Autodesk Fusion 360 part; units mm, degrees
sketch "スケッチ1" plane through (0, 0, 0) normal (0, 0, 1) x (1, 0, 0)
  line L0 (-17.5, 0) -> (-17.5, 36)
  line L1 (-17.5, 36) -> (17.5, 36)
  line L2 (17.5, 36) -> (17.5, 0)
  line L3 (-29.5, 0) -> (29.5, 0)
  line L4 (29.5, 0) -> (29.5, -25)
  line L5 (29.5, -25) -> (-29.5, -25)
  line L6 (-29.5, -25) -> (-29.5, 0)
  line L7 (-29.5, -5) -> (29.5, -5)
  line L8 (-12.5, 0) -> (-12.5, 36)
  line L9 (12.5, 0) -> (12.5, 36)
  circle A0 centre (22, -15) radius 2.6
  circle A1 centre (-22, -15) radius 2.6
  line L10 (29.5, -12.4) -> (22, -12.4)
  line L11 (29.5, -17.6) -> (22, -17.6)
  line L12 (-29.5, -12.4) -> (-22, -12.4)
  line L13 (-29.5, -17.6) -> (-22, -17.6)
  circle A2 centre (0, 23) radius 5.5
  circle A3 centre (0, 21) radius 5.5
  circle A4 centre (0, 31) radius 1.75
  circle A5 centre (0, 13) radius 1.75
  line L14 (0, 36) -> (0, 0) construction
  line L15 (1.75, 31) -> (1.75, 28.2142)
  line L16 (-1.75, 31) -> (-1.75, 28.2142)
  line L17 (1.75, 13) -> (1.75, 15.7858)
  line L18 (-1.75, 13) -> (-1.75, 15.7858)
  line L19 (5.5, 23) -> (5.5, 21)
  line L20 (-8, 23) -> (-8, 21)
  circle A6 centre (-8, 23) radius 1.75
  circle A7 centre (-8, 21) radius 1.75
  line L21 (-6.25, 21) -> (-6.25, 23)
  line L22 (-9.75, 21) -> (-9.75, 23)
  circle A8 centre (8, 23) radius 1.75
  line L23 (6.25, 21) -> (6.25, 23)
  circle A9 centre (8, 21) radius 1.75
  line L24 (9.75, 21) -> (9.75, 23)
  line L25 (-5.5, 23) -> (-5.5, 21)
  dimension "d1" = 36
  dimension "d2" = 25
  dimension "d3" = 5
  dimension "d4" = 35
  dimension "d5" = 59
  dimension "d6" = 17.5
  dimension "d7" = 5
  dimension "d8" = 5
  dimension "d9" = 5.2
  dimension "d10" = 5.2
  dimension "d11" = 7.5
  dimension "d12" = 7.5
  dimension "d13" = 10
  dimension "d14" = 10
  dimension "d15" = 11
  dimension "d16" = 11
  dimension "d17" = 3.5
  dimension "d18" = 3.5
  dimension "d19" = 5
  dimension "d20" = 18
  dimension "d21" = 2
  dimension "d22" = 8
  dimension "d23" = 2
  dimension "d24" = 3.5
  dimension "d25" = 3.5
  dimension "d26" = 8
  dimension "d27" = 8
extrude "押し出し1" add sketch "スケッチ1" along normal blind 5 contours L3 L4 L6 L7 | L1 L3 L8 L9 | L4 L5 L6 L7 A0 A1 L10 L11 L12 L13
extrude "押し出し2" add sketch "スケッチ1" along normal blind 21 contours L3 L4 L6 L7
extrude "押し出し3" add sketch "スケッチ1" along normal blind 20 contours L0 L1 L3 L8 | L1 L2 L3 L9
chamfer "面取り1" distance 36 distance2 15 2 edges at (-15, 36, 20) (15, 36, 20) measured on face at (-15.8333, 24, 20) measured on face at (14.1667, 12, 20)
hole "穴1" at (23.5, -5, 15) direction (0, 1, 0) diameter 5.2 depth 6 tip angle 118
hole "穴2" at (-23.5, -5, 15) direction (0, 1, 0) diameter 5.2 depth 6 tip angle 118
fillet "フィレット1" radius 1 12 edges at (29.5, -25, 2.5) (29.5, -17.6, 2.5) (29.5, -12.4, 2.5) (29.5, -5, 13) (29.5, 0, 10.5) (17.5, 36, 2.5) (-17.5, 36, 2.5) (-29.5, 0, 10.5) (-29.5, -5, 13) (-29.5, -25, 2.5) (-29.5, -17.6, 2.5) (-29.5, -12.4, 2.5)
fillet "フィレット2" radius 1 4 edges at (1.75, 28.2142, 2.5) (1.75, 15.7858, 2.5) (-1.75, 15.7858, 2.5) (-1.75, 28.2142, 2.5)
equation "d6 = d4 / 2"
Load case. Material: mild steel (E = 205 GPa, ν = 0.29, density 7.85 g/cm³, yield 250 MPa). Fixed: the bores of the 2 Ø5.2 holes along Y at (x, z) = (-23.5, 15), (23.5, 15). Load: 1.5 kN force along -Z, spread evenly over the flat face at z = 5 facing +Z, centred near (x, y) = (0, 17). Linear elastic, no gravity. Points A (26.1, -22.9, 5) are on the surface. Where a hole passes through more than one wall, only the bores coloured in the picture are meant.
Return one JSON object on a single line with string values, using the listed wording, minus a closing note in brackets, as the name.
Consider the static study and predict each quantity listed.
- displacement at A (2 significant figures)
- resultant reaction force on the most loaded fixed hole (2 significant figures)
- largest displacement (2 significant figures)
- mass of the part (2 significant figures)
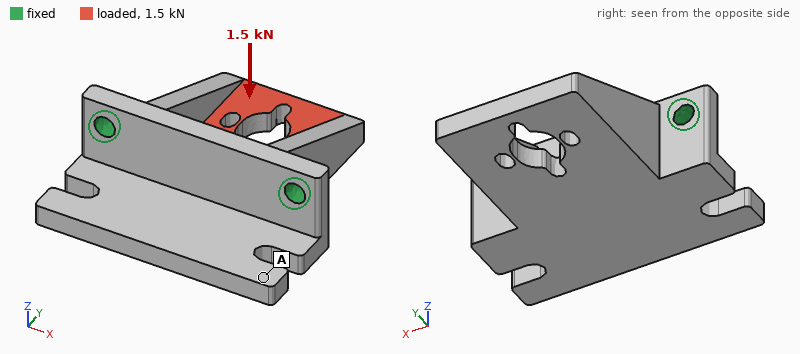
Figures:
{"displacement at A": "34 µm", "resultant reaction force on the most loaded fixed hole": "870 N", "largest displacement": "78 µm", "mass of the part": "150 g"}
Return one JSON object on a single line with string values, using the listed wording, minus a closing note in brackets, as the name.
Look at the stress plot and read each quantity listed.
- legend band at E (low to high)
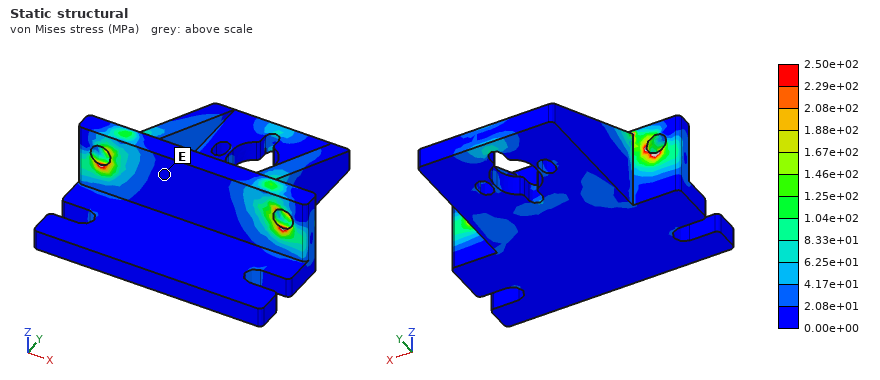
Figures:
{"legend band at E": "0.00e+00 to 2.08e+01 MPa"}
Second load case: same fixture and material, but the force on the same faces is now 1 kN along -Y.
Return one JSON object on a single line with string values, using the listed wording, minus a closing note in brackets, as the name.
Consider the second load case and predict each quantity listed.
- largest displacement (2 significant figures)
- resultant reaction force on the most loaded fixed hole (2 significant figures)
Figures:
{"largest displacement": "17 µm", "resultant reaction force on the most loaded fixed hole": "500 N"}
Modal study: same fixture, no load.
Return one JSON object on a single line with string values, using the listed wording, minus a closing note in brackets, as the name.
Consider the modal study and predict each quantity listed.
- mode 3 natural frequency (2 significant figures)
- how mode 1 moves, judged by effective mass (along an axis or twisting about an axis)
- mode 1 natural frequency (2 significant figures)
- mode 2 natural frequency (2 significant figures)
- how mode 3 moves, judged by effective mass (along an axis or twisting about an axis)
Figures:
{"mode 3 natural frequency": "7100 Hz", "how mode 1 moves, judged by effective mass": "along Y", "mode 1 natural frequency": "3000 Hz", "mode 2 natural frequency": "6000 Hz", "how mode 3 moves, judged by effective mass": "along Z"}
